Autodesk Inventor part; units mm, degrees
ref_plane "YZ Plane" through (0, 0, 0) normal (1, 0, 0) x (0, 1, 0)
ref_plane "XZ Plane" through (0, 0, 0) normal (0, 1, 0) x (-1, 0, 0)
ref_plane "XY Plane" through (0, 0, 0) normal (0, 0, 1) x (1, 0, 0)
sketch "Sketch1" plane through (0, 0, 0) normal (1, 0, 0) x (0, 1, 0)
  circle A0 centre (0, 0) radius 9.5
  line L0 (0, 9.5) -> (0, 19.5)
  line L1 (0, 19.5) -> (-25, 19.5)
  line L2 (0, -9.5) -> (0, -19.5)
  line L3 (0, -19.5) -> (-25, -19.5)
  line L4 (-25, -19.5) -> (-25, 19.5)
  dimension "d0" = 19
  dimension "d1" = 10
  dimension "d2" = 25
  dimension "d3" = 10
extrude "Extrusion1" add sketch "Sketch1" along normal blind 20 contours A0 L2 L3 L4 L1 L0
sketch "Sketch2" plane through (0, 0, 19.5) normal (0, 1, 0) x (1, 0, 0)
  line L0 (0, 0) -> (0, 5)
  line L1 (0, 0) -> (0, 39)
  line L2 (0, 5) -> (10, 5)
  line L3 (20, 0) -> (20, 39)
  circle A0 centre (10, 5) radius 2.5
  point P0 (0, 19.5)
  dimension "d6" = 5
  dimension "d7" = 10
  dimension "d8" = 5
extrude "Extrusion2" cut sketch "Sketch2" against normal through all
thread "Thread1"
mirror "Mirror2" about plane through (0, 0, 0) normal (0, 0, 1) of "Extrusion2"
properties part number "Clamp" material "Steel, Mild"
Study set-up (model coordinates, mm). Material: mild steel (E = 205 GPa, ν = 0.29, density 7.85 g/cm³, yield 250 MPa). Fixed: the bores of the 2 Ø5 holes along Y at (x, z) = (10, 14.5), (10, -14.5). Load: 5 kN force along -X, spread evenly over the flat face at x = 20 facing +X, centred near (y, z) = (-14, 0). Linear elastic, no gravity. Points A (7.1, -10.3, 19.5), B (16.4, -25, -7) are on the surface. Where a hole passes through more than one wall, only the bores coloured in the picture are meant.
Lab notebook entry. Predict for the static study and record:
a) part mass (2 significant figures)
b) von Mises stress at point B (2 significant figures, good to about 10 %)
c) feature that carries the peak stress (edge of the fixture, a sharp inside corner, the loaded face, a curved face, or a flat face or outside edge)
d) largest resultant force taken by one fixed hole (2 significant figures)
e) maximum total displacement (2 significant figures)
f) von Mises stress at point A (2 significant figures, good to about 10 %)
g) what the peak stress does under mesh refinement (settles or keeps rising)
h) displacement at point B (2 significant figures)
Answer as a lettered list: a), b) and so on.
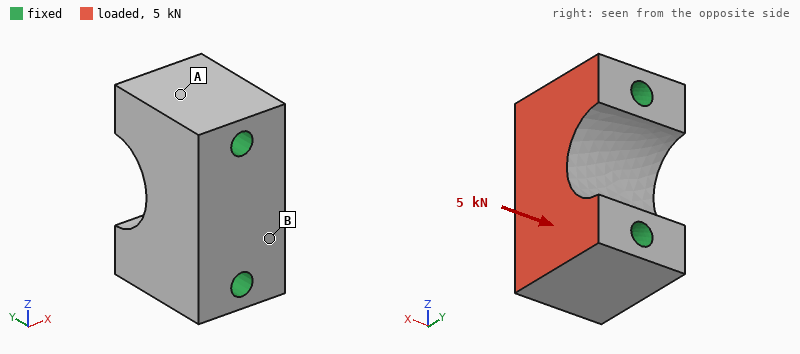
a) 120 g
b) 6.6 MPa
c) edge of the fixture
d) 2.5 kN
e) 0.86 µm
f) 2.4 MPa
g) keeps rising
h) 0.59 µm
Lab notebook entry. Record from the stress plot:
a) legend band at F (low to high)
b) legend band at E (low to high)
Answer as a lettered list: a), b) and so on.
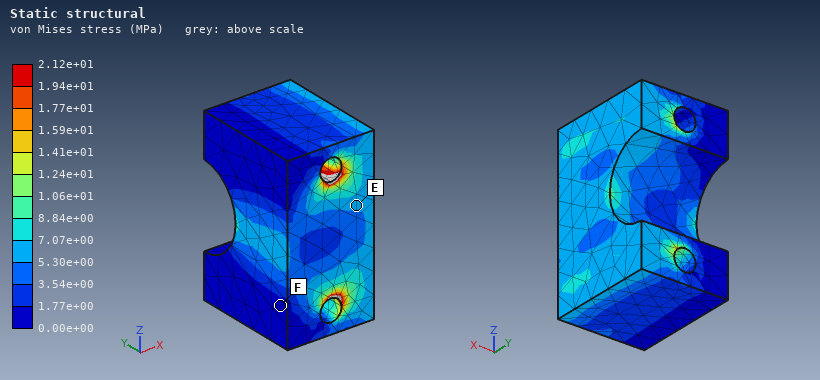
a) 0.00e+00 to 1.77e+00 MPa
b) 5.30e+00 to 7.07e+00 MPa
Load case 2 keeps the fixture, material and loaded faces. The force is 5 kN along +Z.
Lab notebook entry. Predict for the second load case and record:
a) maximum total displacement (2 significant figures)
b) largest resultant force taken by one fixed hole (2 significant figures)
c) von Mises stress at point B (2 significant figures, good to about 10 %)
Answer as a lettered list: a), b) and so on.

a) 1.7 µm
b) 2.8 kN
c) 13 MPa
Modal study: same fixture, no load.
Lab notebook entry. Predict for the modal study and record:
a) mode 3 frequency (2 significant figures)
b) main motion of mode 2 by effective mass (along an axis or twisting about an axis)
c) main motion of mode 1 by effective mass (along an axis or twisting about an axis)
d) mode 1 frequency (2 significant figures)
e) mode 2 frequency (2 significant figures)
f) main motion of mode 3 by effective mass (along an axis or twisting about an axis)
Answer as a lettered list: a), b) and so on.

a) 57 kHz
b) along Y
c) along X
d) 43 kHz
e) 49 kHz
f) twisting about Z
